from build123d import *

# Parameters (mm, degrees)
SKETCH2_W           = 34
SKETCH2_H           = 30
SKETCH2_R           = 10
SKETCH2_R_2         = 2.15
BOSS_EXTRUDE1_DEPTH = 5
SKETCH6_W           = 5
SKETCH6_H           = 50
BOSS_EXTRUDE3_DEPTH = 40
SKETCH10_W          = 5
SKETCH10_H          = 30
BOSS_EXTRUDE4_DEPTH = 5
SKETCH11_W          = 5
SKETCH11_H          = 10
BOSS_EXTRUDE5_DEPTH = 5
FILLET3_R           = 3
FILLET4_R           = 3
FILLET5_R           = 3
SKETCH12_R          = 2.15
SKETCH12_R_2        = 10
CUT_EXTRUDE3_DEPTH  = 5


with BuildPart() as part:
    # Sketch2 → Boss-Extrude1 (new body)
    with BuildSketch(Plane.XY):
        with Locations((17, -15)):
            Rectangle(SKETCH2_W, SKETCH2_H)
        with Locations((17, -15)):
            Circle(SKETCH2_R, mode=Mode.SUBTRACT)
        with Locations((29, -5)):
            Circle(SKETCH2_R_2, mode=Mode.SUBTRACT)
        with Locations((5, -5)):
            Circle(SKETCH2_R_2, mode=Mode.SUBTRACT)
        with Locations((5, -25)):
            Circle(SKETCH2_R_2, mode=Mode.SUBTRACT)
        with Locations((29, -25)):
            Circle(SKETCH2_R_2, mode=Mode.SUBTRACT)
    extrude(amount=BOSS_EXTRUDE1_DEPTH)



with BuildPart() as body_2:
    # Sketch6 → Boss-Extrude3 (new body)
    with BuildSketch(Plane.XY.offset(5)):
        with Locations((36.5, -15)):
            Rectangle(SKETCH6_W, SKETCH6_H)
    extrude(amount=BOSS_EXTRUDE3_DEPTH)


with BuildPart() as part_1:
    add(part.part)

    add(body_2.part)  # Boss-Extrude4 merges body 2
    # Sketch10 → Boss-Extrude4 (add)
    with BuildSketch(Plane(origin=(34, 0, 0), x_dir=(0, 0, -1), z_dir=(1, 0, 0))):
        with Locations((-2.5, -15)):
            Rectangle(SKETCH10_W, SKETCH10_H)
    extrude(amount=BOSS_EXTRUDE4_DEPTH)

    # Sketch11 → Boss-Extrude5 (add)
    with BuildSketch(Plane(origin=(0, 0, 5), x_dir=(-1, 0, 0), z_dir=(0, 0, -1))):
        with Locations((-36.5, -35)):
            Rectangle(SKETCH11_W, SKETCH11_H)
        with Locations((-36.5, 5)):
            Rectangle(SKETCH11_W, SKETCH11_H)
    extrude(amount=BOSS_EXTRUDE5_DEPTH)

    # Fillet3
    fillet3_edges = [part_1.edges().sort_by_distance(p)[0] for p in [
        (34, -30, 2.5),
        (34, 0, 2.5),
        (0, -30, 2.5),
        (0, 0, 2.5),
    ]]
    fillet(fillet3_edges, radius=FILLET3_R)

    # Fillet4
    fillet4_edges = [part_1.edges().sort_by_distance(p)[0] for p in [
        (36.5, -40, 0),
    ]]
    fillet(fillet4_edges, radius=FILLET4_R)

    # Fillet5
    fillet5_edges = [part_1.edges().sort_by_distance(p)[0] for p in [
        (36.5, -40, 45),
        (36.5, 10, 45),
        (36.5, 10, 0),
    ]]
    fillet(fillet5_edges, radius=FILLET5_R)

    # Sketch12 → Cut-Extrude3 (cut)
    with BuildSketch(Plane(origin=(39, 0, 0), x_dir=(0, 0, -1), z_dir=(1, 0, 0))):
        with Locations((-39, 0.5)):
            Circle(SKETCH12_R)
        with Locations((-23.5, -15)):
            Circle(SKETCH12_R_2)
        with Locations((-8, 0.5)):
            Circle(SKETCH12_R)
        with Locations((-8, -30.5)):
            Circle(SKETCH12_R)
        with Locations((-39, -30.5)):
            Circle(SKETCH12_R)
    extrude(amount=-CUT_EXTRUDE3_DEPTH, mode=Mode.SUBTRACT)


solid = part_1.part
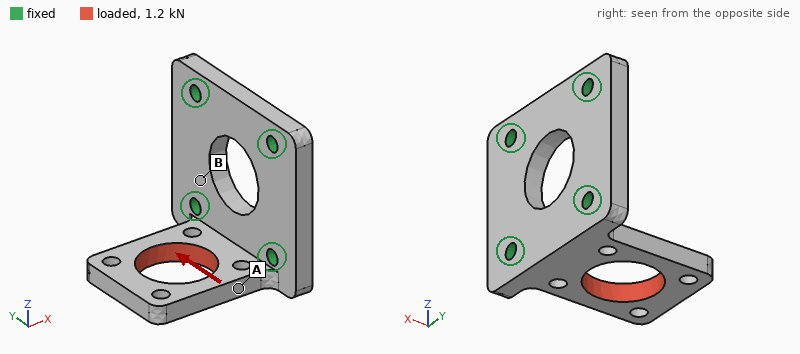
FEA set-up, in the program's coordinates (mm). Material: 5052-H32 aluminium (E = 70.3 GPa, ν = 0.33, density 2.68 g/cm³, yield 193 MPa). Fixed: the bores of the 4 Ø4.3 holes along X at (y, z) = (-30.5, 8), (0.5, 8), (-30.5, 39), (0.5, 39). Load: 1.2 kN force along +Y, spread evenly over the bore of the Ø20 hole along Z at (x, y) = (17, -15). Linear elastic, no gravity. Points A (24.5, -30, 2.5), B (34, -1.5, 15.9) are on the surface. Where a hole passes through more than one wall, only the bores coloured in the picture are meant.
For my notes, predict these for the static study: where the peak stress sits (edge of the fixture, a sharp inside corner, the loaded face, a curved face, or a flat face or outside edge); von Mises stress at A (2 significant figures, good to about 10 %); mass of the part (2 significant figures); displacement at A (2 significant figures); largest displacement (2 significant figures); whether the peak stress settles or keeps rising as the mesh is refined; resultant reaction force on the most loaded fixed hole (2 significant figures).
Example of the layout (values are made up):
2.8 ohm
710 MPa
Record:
edge of the fixture
59 MPa
34 g
19 µm
64 µm
keeps rising
1000 N
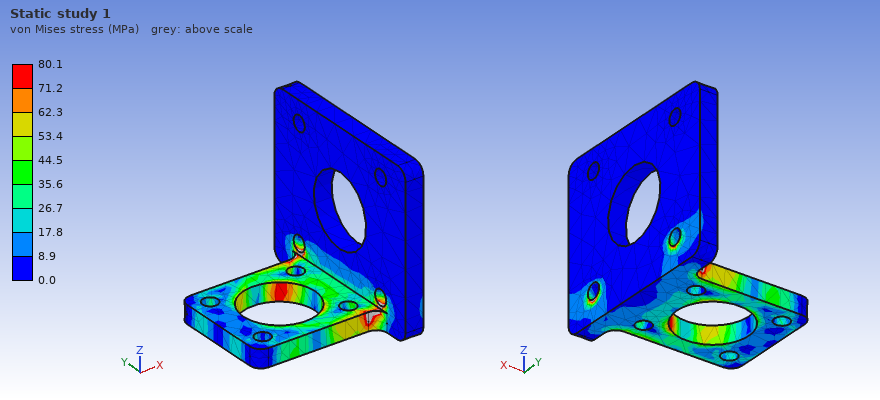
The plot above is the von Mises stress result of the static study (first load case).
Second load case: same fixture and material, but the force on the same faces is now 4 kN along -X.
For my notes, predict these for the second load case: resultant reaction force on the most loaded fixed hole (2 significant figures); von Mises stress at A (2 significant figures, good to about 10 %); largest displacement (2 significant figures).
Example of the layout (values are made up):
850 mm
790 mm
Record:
2.1 kN
71 MPa
0.12 mm
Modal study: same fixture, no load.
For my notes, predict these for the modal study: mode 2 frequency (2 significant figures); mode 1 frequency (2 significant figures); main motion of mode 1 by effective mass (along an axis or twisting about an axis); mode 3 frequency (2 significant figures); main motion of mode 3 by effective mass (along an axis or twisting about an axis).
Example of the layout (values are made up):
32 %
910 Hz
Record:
6300 Hz
2500 Hz
along Z
8300 Hz
along Y
